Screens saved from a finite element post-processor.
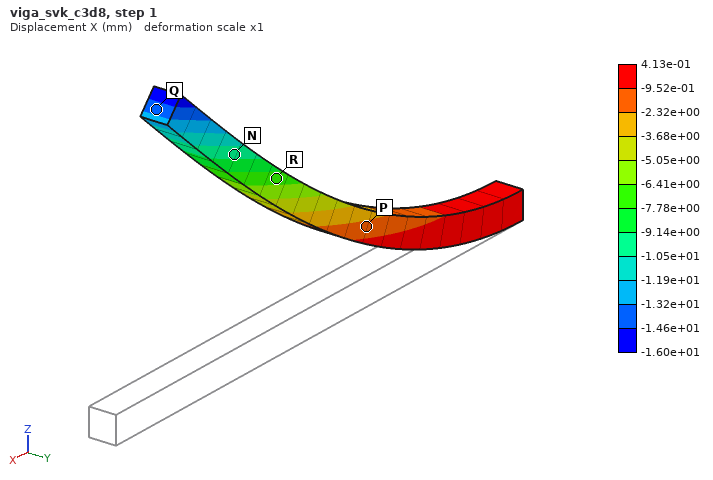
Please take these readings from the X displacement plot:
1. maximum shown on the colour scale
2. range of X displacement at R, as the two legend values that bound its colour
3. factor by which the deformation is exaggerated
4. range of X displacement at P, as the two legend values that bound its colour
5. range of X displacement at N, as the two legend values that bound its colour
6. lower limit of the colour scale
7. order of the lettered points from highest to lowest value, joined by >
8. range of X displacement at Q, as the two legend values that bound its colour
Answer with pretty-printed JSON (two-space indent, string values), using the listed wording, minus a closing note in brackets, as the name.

{
  "maximum shown on the colour scale": "4.13e-01 mm",
  "range of X displacement at R, as the two legend values that bound its colour": "-7.78e+00 to -6.41e+00 mm",
  "factor by which the deformation is exaggerated": "1",
  "range of X displacement at P, as the two legend values that bound its colour": "-2.32e+00 to -9.52e-01 mm",
  "range of X displacement at N, as the two legend values that bound its colour": "-1.05e+01 to -9.14e+00 mm",
  "lower limit of the colour scale": "-1.60e+01 mm",
  "order of the lettered points from highest to lowest value, joined by >": "P > R > N > Q",
  "range of X displacement at Q, as the two legend values that bound its colour": "-1.46e+01 to -1.32e+01 mm"
}
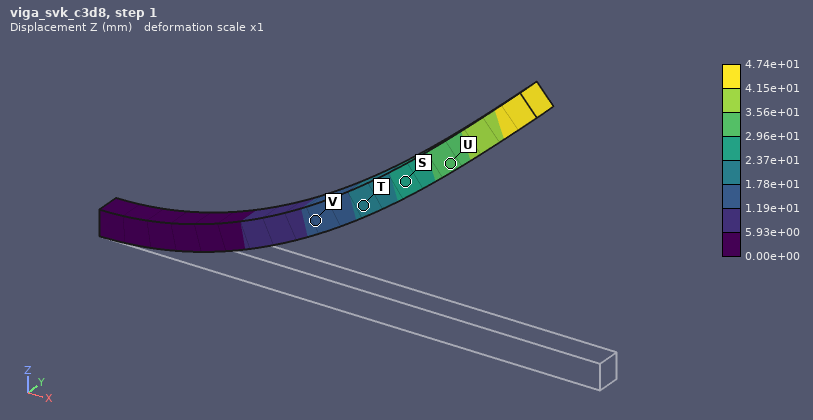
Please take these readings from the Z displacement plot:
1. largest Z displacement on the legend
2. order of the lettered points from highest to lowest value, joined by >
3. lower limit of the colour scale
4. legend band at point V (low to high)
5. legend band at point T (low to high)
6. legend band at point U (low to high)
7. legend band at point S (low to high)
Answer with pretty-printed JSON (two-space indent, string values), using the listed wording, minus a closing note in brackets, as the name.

{
  "largest Z displacement on the legend": "4.74e+01 mm",
  "order of the lettered points from highest to lowest value, joined by >": "U > S > T > V",
  "lower limit of the colour scale": "0.00e+00 mm",
  "legend band at point V": "1.19e+01 to 1.78e+01 mm",
  "legend band at point T": "1.78e+01 to 2.37e+01 mm",
  "legend band at point U": "2.96e+01 to 3.56e+01 mm",
  "legend band at point S": "2.37e+01 to 2.96e+01 mm"
}
